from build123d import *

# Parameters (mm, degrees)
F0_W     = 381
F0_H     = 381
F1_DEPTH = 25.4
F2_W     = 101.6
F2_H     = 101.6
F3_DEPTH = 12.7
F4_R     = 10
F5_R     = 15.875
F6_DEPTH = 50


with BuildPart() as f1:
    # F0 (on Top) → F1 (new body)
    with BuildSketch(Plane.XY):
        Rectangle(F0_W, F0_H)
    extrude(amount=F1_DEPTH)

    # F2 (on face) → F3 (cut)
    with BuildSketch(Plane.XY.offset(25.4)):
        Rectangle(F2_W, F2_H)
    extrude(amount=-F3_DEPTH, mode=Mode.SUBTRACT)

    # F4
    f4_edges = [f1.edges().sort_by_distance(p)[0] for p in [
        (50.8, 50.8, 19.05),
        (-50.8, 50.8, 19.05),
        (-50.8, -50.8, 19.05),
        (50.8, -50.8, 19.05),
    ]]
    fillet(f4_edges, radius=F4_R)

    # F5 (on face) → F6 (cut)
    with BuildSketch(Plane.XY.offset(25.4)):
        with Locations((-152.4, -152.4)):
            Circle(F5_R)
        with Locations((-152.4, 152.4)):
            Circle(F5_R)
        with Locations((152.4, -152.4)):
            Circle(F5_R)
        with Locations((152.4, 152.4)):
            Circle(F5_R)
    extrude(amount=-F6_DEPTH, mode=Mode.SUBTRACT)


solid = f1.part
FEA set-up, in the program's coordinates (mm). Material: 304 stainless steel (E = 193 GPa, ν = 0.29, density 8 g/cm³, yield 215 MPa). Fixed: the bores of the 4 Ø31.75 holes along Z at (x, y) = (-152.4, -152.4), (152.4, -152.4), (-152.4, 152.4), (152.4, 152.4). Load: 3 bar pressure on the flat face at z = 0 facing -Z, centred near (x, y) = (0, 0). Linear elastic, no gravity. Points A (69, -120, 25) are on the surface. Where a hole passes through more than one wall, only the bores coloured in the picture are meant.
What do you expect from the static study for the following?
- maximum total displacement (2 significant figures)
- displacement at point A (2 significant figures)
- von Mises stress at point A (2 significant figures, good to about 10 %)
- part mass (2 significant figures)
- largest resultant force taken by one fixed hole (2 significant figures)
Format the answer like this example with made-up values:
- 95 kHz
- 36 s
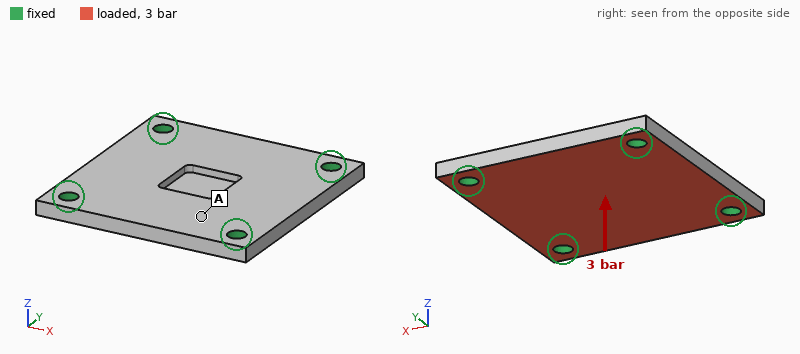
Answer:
- 74 µm
- 30 µm
- 7.1 MPa
- 28 kg
- 11 kN
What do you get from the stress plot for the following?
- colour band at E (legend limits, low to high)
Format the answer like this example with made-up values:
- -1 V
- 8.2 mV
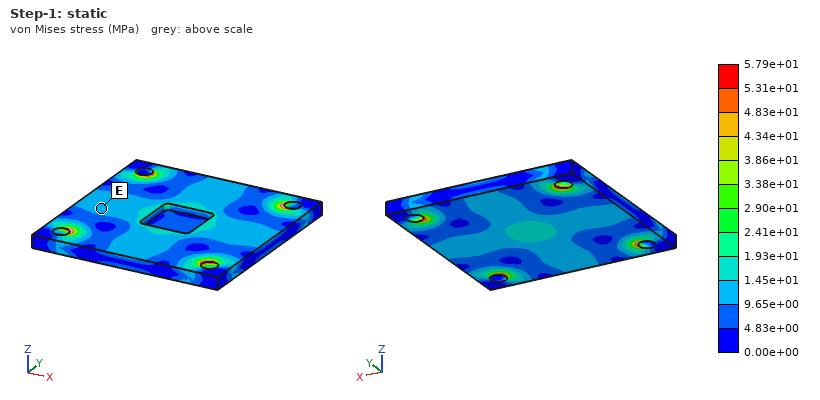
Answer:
- 9.65e+00 to 1.45e+01 MPa
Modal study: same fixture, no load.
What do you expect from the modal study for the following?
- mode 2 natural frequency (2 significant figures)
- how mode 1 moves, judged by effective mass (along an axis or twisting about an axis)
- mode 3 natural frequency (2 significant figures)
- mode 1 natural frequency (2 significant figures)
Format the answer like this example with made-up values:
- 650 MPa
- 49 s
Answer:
- 1600 Hz
- along Z
- 1600 Hz
- 980 Hz
